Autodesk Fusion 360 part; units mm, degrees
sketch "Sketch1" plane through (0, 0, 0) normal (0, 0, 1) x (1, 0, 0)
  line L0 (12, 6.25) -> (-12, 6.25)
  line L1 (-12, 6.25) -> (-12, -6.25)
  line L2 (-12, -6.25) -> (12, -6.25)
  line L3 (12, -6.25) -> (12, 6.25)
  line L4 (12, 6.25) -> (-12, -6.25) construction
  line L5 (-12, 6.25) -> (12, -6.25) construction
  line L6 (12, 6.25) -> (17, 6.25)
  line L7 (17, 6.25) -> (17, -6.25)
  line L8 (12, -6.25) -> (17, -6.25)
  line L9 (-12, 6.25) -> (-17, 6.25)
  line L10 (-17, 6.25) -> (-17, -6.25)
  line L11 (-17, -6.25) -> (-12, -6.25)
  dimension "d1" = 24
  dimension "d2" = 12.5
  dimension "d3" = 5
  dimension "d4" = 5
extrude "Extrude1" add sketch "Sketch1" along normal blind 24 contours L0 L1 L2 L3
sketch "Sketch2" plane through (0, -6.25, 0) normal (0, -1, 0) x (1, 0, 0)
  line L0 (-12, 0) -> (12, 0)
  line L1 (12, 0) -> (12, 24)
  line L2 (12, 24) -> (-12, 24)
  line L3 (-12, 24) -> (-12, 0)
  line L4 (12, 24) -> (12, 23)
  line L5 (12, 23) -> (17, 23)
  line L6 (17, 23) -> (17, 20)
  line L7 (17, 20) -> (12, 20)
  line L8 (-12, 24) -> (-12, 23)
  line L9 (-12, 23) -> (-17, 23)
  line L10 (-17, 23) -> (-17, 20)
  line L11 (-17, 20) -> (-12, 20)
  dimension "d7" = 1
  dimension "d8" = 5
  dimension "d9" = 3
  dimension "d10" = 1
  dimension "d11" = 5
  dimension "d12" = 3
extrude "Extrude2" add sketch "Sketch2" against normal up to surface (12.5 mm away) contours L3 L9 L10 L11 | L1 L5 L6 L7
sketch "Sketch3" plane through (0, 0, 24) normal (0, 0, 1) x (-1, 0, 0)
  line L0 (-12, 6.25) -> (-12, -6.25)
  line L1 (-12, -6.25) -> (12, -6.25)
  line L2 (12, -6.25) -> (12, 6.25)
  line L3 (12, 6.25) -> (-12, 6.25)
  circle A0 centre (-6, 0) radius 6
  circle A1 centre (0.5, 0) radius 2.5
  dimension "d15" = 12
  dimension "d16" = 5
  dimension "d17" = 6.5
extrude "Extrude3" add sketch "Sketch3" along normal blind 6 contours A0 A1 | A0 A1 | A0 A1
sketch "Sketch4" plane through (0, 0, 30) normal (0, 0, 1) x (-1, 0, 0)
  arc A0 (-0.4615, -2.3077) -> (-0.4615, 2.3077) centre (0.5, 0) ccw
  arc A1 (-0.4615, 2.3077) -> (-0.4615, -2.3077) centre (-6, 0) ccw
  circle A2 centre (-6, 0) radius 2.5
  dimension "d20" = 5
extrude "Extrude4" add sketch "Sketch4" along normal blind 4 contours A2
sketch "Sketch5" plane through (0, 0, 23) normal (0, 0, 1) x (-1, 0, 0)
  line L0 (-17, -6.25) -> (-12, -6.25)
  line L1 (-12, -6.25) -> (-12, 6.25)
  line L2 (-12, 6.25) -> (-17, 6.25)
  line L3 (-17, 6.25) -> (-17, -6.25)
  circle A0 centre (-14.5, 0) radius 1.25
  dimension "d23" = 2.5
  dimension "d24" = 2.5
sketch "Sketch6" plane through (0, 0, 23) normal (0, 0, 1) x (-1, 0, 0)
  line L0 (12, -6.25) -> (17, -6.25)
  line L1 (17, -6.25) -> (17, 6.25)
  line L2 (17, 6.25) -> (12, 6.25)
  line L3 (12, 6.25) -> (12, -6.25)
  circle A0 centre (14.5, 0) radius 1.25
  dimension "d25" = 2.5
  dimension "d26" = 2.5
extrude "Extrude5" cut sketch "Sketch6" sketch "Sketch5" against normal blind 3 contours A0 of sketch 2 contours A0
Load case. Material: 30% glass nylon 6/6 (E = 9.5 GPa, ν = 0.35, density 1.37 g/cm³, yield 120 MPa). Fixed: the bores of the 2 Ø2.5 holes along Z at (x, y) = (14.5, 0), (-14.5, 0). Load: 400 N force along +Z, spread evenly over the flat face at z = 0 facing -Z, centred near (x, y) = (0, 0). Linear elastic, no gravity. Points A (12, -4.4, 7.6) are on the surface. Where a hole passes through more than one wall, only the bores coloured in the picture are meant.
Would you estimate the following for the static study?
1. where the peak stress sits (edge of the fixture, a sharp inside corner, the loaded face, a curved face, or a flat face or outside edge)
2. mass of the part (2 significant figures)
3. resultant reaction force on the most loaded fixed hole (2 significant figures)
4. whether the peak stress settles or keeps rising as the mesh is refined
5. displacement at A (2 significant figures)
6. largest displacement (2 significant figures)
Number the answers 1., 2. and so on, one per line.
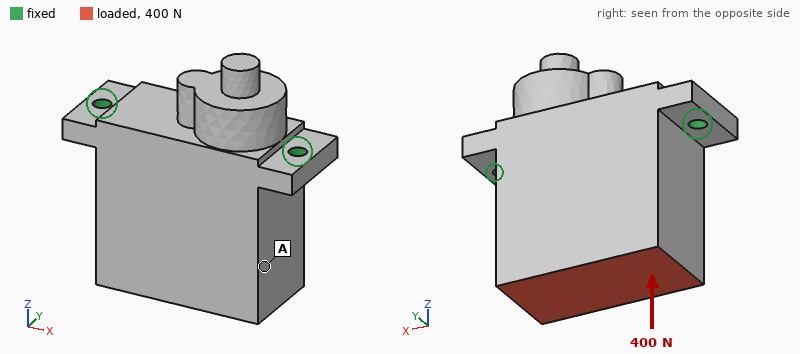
1. edge of the fixture
2. 11 g
3. 210 N
4. keeps rising
5. 14 µm
6. 17 µm
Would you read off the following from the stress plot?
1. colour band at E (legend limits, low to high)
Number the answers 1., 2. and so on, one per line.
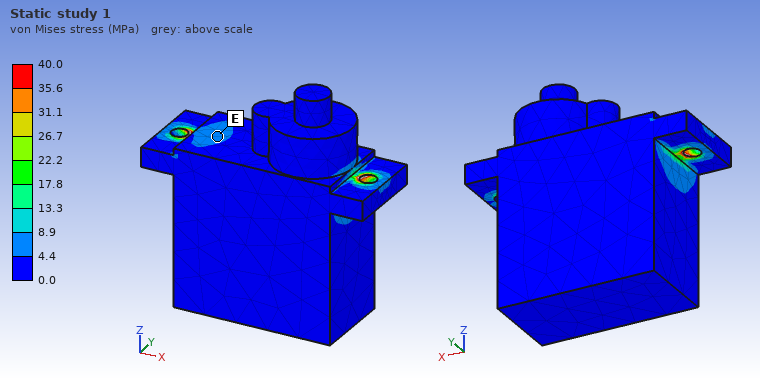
1. 4.4 to 8.9 MPa
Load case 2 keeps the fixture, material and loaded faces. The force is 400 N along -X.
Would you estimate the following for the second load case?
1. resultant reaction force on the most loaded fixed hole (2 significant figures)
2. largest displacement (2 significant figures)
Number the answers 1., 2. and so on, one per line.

1. 390 N
2. 57 µm
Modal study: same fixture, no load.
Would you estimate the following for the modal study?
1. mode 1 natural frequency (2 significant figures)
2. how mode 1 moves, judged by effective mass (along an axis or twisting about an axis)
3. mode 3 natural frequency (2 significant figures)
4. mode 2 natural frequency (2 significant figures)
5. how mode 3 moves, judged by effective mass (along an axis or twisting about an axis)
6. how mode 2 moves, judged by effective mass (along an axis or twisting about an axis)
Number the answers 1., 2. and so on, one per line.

1. 1900 Hz
2. along Y
3. 8100 Hz
4. 7500 Hz
5. along Z
6. along X
